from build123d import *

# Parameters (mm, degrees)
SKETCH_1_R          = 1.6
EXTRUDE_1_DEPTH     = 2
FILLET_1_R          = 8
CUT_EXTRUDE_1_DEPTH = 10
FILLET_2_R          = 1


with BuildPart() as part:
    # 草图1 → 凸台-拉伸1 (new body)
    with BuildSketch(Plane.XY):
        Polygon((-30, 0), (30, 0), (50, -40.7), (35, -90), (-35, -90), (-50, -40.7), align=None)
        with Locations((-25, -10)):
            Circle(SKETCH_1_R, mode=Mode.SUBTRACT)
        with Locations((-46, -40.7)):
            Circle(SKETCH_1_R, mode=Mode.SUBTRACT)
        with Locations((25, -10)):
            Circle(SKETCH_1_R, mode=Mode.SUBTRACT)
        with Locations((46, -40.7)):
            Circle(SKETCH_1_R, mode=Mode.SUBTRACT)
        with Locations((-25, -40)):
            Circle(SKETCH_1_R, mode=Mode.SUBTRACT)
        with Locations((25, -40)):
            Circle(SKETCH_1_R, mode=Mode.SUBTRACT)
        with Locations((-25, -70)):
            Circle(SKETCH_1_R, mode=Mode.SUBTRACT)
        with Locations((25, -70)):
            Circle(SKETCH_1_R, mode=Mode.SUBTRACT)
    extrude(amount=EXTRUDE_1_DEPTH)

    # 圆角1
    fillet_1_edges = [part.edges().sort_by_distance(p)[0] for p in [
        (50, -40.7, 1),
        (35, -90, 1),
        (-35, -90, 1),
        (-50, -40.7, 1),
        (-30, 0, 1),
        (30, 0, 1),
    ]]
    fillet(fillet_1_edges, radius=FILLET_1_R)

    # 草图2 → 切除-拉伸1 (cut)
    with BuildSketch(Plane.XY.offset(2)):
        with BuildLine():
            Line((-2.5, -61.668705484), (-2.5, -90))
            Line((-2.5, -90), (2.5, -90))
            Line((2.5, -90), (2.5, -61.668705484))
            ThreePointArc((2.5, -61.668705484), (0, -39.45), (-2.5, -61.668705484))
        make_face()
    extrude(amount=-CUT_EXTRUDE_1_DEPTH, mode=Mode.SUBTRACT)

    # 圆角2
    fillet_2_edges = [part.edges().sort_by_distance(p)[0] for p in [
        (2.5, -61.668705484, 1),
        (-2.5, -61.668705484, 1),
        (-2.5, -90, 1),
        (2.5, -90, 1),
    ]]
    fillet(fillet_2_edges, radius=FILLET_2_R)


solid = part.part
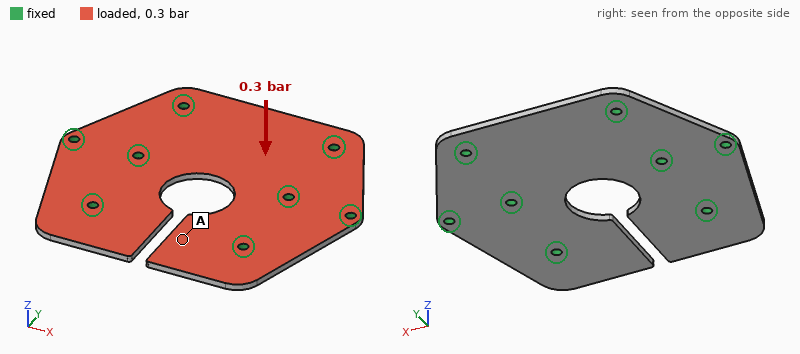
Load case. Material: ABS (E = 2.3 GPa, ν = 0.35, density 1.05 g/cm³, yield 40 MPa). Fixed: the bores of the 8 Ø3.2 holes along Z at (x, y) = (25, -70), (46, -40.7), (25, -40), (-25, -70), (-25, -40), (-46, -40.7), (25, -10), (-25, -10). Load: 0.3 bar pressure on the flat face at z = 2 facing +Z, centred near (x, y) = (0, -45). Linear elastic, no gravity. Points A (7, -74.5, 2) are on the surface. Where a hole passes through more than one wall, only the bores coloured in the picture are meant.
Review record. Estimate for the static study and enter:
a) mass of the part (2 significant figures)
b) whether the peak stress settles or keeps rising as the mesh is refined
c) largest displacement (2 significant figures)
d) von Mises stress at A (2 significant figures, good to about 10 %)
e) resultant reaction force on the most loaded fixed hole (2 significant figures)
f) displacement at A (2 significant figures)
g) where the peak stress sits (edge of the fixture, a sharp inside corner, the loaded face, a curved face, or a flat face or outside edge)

14 g
keeps rising
1.00 mm
2.0 MPa
39 N
0.53 mm
edge of the fixture
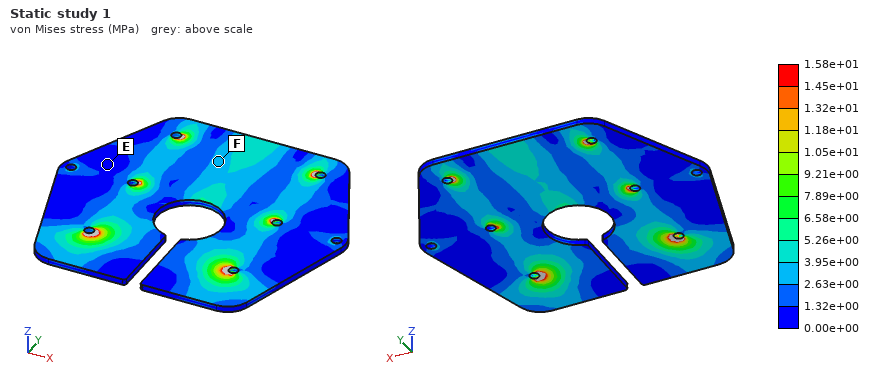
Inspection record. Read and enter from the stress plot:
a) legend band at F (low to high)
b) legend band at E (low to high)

2.63e+00 to 3.95e+00 MPa
0.00e+00 to 1.32e+00 MPa
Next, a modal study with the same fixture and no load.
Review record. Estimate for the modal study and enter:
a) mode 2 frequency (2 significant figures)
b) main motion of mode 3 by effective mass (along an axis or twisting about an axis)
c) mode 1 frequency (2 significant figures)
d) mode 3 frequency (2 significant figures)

810 Hz
along Z
810 Hz
1200 Hz
